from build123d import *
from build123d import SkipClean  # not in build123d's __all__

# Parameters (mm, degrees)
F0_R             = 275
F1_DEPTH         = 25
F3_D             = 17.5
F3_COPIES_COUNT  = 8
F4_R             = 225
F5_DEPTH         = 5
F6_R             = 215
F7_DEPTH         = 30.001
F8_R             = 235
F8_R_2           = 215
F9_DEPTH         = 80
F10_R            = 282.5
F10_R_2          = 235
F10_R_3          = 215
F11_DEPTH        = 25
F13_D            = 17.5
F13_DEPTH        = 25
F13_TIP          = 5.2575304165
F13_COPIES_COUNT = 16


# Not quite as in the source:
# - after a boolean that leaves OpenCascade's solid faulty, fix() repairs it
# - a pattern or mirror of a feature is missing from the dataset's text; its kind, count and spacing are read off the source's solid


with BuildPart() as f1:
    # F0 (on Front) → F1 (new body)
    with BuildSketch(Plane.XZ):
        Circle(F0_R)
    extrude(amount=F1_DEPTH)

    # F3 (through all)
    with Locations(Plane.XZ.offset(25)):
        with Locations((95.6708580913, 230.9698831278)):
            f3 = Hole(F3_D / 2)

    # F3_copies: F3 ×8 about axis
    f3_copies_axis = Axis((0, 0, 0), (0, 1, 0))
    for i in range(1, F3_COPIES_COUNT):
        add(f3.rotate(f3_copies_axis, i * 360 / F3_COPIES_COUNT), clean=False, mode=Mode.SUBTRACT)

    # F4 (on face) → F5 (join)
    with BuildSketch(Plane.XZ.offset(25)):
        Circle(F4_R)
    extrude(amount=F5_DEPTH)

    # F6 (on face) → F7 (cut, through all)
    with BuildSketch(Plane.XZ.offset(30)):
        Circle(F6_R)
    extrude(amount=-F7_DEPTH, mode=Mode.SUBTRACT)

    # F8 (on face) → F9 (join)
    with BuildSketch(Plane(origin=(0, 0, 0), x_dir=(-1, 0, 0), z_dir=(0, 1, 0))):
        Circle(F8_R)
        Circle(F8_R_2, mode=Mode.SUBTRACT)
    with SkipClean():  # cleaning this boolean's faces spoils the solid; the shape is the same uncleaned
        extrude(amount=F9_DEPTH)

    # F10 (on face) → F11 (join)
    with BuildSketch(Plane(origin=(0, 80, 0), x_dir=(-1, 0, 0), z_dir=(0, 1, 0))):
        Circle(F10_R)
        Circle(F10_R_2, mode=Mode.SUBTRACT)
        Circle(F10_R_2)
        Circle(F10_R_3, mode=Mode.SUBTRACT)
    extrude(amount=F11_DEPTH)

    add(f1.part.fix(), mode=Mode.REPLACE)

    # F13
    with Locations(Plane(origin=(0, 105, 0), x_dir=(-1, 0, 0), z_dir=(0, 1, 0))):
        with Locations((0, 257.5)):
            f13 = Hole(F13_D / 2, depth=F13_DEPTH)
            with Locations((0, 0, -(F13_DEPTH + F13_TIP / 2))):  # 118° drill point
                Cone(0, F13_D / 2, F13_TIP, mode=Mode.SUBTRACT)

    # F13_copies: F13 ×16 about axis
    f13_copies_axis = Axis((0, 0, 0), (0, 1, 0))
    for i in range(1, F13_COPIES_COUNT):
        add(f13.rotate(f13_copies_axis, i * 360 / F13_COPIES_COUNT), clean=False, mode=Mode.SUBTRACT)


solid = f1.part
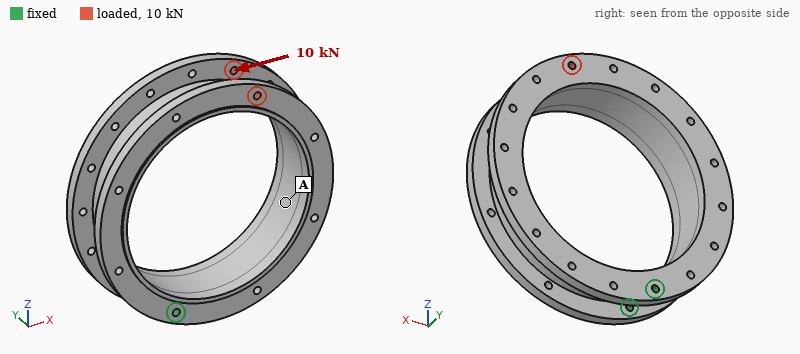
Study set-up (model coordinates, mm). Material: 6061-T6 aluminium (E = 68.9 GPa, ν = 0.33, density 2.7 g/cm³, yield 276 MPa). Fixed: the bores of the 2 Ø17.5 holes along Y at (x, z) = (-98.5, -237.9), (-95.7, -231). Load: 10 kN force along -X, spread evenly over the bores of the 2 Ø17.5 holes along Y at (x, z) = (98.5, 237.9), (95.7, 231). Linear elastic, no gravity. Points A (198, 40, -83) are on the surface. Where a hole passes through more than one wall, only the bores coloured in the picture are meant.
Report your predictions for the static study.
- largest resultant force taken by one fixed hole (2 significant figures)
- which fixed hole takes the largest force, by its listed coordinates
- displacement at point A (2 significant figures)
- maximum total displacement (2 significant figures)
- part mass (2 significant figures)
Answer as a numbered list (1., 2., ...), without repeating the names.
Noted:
1. 7.7 kN
2. (-95.7, -231)
3. 1.9 mm
4. 3.3 mm
5. 19 kg
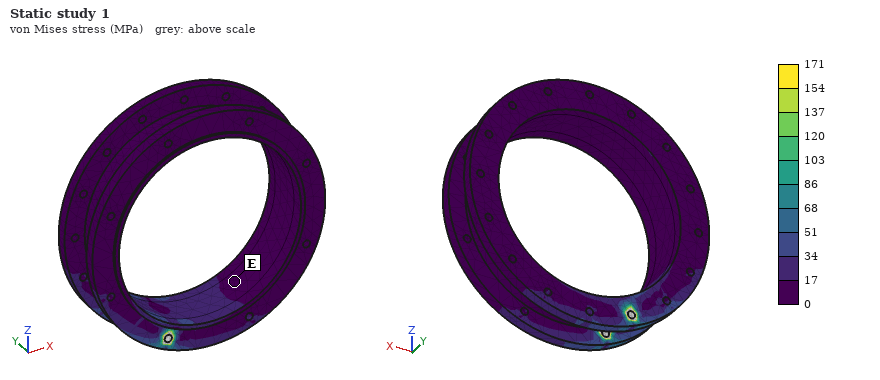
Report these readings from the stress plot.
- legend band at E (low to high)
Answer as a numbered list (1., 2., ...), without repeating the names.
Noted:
1. 0 to 17 MPa
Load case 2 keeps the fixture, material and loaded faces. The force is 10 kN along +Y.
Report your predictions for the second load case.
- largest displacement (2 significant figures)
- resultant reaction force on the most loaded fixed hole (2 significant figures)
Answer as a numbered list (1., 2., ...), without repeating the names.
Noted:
1. 4.6 mm
2. 43 kN
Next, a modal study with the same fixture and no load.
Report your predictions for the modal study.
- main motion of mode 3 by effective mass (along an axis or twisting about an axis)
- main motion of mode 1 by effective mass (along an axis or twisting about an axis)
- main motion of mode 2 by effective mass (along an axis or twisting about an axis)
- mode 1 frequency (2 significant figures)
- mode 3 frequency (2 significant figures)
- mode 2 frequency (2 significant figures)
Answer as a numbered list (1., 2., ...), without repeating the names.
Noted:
1. twisting about Z
2. along X
3. along Y
4. 91 Hz
5. 300 Hz
6. 110 Hz
